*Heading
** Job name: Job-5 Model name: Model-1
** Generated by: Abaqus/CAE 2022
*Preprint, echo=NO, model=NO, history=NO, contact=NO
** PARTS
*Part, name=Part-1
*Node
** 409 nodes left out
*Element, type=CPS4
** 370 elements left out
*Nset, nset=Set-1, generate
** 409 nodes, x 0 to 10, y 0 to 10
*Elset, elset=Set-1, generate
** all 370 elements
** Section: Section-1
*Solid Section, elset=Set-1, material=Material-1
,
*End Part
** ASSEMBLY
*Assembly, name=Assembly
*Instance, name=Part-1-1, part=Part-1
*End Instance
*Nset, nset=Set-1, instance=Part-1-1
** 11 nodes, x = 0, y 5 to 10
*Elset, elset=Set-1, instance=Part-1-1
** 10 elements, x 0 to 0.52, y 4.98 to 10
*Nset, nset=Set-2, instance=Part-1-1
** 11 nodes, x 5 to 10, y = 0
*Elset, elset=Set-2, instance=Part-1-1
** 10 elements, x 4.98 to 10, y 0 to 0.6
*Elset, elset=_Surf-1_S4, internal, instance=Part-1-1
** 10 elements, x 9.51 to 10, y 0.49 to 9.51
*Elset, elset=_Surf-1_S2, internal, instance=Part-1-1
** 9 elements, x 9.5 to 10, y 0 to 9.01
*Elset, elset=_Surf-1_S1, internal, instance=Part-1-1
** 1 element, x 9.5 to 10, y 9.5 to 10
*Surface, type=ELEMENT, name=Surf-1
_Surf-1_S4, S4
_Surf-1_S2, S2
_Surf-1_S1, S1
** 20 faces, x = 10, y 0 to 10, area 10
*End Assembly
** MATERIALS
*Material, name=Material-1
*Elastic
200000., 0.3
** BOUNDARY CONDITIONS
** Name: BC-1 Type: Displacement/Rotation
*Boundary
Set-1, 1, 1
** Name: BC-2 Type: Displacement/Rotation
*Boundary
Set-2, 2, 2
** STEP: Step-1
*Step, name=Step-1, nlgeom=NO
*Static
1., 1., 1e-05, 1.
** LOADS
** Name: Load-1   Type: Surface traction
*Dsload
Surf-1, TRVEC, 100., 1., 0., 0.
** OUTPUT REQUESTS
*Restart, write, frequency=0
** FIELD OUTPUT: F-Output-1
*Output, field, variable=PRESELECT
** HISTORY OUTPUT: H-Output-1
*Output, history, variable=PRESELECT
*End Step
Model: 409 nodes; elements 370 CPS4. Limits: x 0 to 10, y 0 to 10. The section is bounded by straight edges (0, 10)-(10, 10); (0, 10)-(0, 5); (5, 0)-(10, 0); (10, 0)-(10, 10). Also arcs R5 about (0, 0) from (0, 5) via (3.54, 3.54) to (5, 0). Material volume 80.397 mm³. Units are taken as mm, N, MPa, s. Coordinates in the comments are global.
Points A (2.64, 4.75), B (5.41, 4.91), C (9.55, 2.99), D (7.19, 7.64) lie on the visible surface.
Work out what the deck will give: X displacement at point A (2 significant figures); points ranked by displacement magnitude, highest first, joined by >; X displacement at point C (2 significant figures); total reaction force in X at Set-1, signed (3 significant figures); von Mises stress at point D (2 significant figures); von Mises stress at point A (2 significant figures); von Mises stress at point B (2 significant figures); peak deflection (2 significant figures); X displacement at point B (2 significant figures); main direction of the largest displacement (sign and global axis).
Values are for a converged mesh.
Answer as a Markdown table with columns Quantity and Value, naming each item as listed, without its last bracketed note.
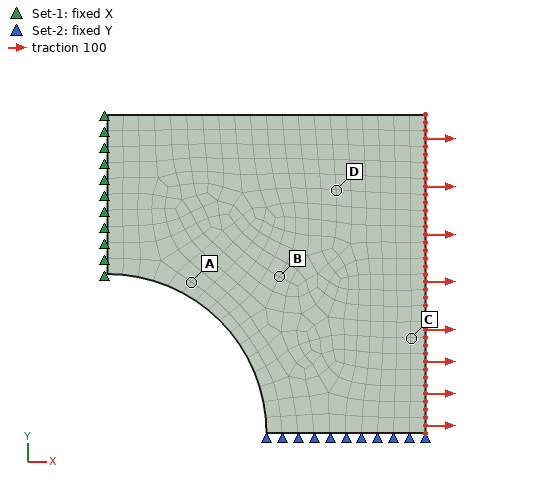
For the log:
| Quantity | Value |
|---|---|
| X displacement at point A | 0.0069 mm |
| points ranked by displacement magnitude, highest first, joined by > | C > A > B > D |
| X displacement at point C | 0.016 mm |
| total reaction force in X at Set-1, signed | -1000 N |
| von Mises stress at point D | 130 MPa |
| von Mises stress at point A | 310 MPa |
| von Mises stress at point B | 220 MPa |
| peak deflection | 0.019 mm |
| X displacement at point B | 0.0096 mm |
| main direction of the largest displacement | +X |
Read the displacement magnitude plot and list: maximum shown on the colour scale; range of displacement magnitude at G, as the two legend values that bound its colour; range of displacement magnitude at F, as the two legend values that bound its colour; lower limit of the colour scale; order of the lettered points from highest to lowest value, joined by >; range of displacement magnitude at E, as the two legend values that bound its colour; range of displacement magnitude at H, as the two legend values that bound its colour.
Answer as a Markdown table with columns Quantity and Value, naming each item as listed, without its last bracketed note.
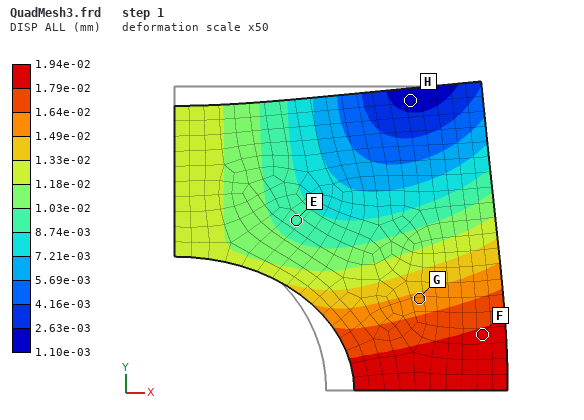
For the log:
| Quantity | Value |
|---|---|
| maximum shown on the colour scale | 1.94e-02 mm |
| range of displacement magnitude at G, as the two legend values that bound its colour | 1.49e-02 to 1.64e-02 mm |
| range of displacement magnitude at F, as the two legend values that bound its colour | 1.79e-02 to 1.94e-02 mm |
| lower limit of the colour scale | 1.10e-03 mm |
| order of the lettered points from highest to lowest value, joined by > | F > G > E > H |
| range of displacement magnitude at E, as the two legend values that bound its colour | 8.74e-03 to 1.03e-02 mm |
| range of displacement magnitude at H, as the two legend values that bound its colour | 1.10e-03 to 2.63e-03 mm |
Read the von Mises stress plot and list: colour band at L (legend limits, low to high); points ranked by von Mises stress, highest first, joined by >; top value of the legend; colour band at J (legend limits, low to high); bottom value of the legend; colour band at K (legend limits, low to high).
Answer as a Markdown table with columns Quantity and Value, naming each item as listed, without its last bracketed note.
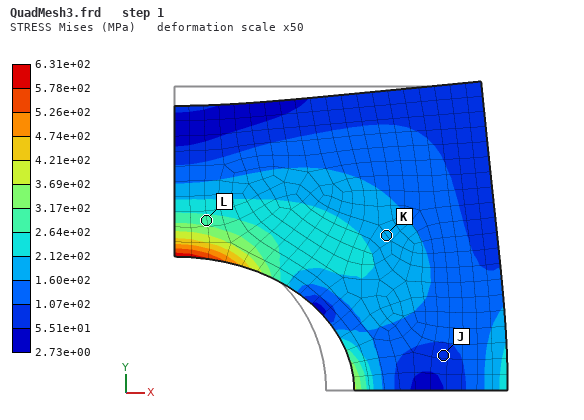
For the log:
| Quantity | Value |
|---|---|
| colour band at L | 2.64e+02 to 3.17e+02 MPa |
| points ranked by von Mises stress, highest first, joined by > | L > K > J |
| top value of the legend | 6.31e+02 MPa |
| colour band at J | 5.51e+01 to 1.07e+02 MPa |
| bottom value of the legend | 2.73e+00 MPa |
| colour band at K | 1.60e+02 to 2.12e+02 MPa |
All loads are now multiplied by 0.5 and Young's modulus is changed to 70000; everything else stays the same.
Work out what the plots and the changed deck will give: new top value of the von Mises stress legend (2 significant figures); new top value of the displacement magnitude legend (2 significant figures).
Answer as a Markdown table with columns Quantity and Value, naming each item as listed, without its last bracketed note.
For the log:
| Quantity | Value |
|---|---|
| new top value of the von Mises stress legend | 320 MPa |
| new top value of the displacement magnitude legend | 0.028 mm |
